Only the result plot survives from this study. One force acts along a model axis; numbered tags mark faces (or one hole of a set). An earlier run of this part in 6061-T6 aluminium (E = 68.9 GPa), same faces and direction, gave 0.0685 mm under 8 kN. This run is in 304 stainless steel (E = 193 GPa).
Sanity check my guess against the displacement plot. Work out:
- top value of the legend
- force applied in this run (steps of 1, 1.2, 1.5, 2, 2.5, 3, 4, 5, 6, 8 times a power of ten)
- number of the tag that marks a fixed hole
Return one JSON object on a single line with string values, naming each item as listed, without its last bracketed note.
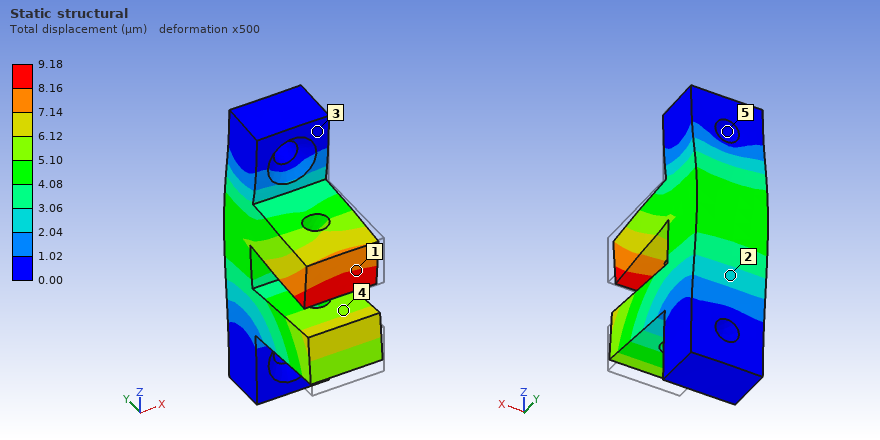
{"top value of the legend": "9.18 µm", "force applied in this run": "3 kN", "number of the tag that marks a fixed hole": "5"}
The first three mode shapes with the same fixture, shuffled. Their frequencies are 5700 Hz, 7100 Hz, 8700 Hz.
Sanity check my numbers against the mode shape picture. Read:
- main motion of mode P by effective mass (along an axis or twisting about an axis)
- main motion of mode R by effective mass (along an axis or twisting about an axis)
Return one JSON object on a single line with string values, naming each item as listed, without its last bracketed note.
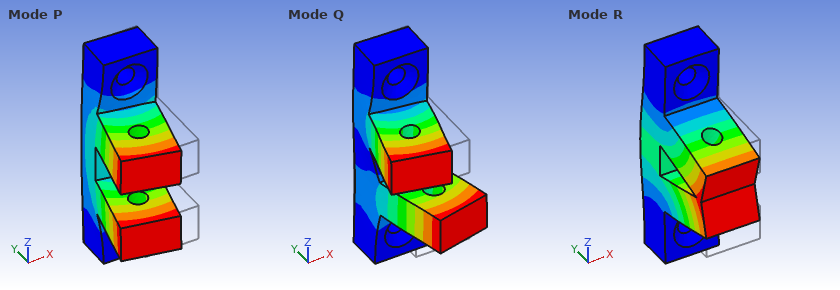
{"main motion of mode P by effective mass": "along X", "main motion of mode R by effective mass": "along Y"}
